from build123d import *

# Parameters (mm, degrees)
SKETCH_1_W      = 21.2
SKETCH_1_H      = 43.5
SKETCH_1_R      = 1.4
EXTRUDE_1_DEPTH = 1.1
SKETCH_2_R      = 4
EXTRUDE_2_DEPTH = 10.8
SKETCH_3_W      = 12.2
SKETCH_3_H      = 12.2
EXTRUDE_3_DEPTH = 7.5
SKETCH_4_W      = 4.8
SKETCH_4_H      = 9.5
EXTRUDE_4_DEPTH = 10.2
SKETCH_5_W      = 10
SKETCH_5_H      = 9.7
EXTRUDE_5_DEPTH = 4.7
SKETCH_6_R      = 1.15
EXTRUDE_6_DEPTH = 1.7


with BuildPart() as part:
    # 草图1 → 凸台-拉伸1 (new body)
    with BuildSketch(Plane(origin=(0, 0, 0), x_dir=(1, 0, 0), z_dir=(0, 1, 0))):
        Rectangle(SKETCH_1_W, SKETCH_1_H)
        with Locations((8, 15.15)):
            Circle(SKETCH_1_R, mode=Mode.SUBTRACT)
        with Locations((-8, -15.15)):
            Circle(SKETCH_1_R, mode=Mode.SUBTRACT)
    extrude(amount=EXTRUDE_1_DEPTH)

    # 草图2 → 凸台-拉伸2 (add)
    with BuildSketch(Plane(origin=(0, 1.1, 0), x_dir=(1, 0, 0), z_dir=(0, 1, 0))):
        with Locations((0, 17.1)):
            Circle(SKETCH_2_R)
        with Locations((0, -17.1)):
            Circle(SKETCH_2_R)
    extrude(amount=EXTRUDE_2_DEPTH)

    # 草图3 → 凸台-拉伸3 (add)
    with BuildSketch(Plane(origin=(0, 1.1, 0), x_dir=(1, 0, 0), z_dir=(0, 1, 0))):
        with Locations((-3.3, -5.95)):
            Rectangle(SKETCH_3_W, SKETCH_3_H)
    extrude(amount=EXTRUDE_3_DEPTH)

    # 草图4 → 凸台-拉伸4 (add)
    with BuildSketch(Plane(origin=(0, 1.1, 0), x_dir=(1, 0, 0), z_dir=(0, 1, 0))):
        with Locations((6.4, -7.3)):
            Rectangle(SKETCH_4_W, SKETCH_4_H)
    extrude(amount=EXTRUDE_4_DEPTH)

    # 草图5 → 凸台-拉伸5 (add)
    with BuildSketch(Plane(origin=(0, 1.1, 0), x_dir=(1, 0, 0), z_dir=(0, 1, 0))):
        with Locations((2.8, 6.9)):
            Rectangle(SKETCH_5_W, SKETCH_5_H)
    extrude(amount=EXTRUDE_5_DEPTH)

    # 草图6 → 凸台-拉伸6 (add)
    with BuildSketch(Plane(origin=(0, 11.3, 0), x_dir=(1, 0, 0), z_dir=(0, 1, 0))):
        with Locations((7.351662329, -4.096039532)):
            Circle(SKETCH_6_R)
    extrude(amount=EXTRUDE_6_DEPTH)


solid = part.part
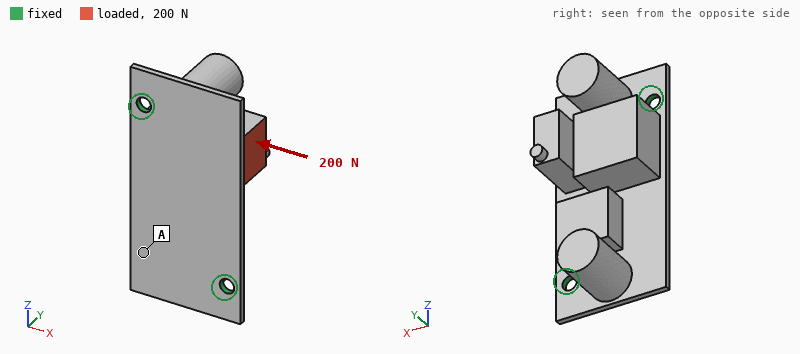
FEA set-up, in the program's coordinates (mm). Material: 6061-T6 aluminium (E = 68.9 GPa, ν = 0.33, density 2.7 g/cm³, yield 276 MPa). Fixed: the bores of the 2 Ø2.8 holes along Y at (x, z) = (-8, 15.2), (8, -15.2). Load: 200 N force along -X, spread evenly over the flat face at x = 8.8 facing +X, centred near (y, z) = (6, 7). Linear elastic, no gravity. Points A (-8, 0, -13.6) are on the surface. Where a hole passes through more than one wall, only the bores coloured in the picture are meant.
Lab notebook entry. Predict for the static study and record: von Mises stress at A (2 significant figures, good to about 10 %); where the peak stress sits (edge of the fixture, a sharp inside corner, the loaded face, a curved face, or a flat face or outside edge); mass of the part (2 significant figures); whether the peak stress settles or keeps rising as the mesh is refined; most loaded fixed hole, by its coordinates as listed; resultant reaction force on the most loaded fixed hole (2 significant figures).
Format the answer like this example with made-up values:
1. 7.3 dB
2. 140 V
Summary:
1. 20 MPa
2. edge of the fixture
3. 11 g
4. keeps rising
5. (-8, 15.2)
6. 140 N
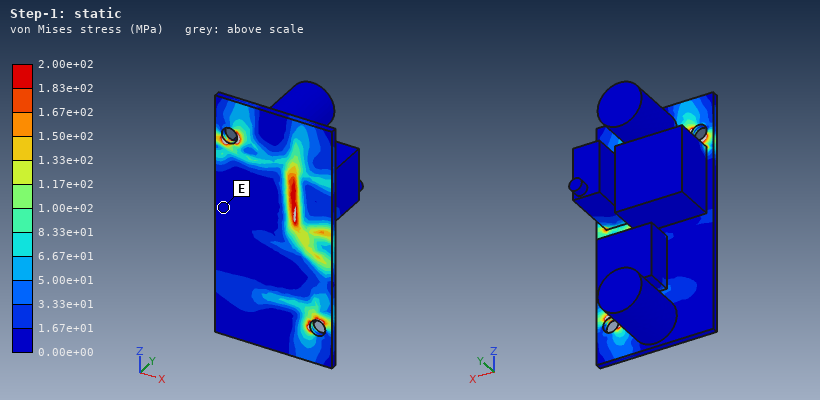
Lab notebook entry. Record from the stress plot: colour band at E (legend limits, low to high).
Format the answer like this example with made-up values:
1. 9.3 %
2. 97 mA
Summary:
1. 0.00e+00 to 1.67e+01 MPa
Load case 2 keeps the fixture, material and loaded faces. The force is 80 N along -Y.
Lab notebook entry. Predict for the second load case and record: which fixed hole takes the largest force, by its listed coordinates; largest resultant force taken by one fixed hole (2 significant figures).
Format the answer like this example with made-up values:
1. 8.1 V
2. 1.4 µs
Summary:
1. (-8, 15.2)
2. 58 N
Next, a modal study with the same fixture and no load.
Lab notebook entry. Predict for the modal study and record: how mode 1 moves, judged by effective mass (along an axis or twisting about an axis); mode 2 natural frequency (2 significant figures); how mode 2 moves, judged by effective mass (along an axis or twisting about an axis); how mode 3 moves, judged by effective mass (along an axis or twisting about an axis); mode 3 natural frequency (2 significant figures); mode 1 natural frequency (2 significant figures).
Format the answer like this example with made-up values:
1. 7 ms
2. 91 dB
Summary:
1. along X
2. 2900 Hz
3. along Y
4. along Y
5. 3600 Hz
6. 2000 Hz
